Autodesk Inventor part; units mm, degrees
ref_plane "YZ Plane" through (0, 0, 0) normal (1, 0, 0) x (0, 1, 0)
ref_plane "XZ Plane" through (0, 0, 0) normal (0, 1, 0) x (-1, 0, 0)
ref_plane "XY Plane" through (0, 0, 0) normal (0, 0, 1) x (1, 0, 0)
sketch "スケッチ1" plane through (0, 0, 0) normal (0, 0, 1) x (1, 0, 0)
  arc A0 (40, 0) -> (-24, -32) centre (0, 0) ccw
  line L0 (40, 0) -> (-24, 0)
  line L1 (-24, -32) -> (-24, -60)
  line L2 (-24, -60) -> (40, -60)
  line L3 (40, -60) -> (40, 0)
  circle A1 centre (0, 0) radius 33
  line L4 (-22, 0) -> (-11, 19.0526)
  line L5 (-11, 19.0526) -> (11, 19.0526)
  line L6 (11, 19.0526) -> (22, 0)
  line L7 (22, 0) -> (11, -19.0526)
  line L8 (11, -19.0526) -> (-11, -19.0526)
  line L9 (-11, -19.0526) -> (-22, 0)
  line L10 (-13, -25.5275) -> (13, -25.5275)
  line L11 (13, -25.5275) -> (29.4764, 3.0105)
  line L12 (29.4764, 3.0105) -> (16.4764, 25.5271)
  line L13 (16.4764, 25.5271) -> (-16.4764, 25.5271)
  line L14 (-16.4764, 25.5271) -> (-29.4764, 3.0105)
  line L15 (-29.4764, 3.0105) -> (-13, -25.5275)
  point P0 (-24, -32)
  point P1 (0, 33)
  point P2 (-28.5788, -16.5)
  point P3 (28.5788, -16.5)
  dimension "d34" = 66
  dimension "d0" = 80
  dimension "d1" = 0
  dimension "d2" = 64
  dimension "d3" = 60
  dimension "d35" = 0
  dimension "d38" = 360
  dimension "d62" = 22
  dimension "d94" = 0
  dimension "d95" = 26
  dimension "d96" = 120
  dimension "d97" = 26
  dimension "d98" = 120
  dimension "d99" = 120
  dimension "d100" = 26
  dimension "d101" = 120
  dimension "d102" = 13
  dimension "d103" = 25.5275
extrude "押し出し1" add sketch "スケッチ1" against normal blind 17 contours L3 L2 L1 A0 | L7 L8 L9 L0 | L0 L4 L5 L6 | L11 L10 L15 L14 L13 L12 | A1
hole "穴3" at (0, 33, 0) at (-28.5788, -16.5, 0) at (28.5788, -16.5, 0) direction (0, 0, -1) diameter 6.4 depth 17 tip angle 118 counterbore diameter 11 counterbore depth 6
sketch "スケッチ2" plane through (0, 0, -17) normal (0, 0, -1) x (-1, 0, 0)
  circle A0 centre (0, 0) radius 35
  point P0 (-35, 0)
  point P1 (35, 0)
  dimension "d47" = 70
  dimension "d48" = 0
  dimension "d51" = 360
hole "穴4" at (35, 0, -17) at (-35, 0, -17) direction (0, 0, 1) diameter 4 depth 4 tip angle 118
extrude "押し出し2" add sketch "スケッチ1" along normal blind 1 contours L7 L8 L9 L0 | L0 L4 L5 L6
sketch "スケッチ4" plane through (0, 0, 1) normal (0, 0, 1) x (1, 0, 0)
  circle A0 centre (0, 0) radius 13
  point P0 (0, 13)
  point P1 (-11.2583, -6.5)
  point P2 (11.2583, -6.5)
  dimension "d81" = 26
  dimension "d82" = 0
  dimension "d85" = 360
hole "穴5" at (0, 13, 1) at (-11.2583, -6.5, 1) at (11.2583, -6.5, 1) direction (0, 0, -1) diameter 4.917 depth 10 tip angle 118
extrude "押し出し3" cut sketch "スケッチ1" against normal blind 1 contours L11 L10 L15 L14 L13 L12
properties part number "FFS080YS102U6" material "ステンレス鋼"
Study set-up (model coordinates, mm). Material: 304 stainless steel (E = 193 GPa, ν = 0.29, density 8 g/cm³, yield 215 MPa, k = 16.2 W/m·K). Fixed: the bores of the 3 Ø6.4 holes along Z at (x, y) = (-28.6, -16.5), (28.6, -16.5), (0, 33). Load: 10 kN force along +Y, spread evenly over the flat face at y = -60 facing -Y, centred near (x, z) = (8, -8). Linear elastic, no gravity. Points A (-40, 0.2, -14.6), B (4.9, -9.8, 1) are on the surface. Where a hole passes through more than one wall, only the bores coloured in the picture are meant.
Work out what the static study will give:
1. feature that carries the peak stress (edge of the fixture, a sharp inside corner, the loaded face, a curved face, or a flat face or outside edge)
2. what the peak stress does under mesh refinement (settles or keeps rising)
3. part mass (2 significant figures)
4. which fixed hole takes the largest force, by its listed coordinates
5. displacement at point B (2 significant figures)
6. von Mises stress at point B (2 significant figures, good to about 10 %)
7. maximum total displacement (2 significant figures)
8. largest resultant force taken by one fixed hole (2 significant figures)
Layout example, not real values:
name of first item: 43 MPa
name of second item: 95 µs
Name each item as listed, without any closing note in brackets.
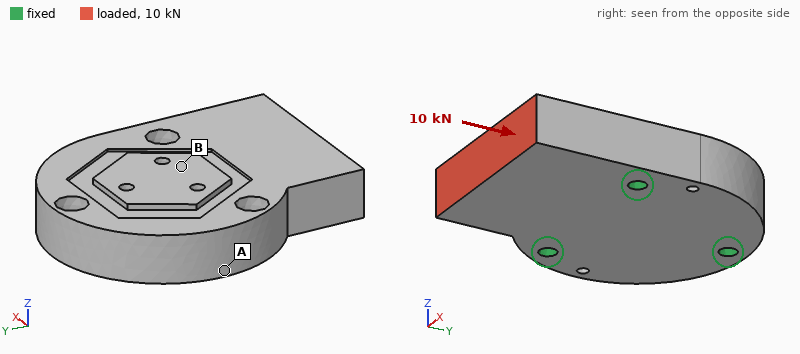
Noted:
feature that carries the peak stress: edge of the fixture
what the peak stress does under mesh refinement: keeps rising
part mass: 890 g
which fixed hole takes the largest force, by its listed coordinates: (28.6, -16.5)
displacement at point B: 1.4 µm
von Mises stress at point B: 7.5 MPa
maximum total displacement: 4.7 µm
largest resultant force taken by one fixed hole: 5.4 kN
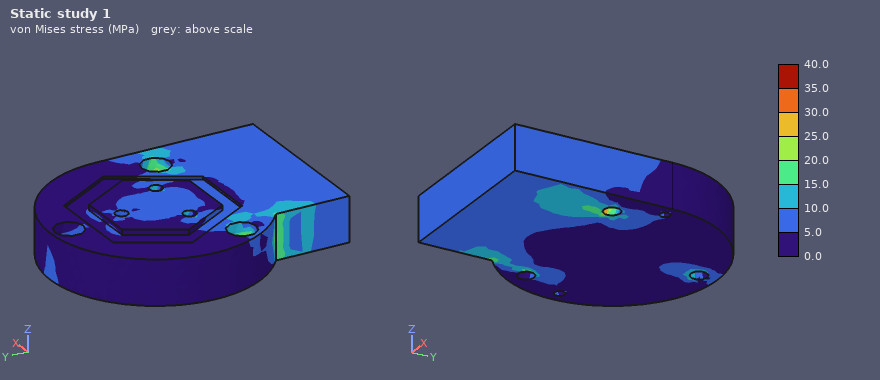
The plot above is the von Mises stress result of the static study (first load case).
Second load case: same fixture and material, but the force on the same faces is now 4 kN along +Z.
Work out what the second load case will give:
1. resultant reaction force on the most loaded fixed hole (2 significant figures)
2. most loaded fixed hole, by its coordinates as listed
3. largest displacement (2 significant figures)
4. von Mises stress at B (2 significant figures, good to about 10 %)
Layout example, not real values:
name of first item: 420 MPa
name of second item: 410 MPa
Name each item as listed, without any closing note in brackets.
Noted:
resultant reaction force on the most loaded fixed hole: 3.7 kN
most loaded fixed hole, by its coordinates as listed: (28.6, -16.5)
largest displacement: 43 µm
von Mises stress at B: 33 MPa
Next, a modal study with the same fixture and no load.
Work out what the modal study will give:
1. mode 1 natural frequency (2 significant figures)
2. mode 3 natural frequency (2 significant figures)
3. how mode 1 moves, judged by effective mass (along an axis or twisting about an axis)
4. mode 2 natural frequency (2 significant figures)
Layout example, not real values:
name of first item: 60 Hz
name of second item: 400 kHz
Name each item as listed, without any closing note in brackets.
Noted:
mode 1 natural frequency: 4600 Hz
mode 3 natural frequency: 11 kHz
how mode 1 moves, judged by effective mass: along Z
mode 2 natural frequency: 9500 Hz
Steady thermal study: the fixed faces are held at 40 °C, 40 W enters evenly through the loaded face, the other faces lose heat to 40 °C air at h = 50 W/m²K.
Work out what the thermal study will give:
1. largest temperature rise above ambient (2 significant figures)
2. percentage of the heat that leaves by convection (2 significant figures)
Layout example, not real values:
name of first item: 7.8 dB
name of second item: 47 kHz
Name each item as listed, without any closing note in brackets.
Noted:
largest temperature rise above ambient: 86 K
percentage of the heat that leaves by convection: 46 %
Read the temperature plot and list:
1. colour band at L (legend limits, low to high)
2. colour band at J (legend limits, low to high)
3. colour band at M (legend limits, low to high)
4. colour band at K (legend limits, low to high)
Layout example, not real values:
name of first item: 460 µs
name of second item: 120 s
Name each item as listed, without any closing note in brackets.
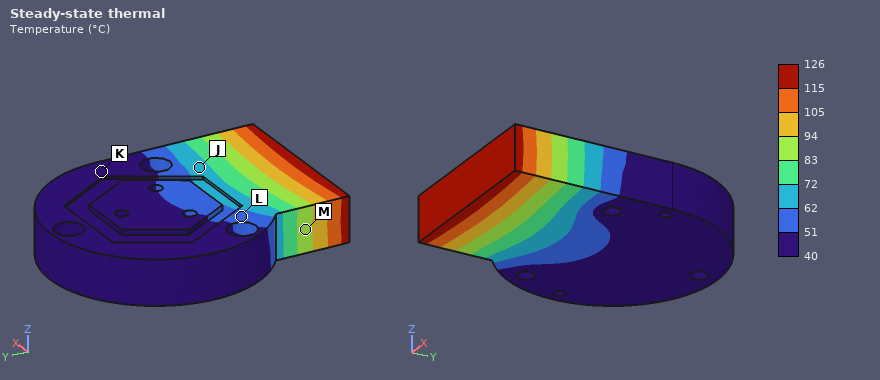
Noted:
colour band at L: 51 to 62 °C
colour band at J: 62 to 72 °C
colour band at M: 83 to 94 °C
colour band at K: 40 to 51 °C
